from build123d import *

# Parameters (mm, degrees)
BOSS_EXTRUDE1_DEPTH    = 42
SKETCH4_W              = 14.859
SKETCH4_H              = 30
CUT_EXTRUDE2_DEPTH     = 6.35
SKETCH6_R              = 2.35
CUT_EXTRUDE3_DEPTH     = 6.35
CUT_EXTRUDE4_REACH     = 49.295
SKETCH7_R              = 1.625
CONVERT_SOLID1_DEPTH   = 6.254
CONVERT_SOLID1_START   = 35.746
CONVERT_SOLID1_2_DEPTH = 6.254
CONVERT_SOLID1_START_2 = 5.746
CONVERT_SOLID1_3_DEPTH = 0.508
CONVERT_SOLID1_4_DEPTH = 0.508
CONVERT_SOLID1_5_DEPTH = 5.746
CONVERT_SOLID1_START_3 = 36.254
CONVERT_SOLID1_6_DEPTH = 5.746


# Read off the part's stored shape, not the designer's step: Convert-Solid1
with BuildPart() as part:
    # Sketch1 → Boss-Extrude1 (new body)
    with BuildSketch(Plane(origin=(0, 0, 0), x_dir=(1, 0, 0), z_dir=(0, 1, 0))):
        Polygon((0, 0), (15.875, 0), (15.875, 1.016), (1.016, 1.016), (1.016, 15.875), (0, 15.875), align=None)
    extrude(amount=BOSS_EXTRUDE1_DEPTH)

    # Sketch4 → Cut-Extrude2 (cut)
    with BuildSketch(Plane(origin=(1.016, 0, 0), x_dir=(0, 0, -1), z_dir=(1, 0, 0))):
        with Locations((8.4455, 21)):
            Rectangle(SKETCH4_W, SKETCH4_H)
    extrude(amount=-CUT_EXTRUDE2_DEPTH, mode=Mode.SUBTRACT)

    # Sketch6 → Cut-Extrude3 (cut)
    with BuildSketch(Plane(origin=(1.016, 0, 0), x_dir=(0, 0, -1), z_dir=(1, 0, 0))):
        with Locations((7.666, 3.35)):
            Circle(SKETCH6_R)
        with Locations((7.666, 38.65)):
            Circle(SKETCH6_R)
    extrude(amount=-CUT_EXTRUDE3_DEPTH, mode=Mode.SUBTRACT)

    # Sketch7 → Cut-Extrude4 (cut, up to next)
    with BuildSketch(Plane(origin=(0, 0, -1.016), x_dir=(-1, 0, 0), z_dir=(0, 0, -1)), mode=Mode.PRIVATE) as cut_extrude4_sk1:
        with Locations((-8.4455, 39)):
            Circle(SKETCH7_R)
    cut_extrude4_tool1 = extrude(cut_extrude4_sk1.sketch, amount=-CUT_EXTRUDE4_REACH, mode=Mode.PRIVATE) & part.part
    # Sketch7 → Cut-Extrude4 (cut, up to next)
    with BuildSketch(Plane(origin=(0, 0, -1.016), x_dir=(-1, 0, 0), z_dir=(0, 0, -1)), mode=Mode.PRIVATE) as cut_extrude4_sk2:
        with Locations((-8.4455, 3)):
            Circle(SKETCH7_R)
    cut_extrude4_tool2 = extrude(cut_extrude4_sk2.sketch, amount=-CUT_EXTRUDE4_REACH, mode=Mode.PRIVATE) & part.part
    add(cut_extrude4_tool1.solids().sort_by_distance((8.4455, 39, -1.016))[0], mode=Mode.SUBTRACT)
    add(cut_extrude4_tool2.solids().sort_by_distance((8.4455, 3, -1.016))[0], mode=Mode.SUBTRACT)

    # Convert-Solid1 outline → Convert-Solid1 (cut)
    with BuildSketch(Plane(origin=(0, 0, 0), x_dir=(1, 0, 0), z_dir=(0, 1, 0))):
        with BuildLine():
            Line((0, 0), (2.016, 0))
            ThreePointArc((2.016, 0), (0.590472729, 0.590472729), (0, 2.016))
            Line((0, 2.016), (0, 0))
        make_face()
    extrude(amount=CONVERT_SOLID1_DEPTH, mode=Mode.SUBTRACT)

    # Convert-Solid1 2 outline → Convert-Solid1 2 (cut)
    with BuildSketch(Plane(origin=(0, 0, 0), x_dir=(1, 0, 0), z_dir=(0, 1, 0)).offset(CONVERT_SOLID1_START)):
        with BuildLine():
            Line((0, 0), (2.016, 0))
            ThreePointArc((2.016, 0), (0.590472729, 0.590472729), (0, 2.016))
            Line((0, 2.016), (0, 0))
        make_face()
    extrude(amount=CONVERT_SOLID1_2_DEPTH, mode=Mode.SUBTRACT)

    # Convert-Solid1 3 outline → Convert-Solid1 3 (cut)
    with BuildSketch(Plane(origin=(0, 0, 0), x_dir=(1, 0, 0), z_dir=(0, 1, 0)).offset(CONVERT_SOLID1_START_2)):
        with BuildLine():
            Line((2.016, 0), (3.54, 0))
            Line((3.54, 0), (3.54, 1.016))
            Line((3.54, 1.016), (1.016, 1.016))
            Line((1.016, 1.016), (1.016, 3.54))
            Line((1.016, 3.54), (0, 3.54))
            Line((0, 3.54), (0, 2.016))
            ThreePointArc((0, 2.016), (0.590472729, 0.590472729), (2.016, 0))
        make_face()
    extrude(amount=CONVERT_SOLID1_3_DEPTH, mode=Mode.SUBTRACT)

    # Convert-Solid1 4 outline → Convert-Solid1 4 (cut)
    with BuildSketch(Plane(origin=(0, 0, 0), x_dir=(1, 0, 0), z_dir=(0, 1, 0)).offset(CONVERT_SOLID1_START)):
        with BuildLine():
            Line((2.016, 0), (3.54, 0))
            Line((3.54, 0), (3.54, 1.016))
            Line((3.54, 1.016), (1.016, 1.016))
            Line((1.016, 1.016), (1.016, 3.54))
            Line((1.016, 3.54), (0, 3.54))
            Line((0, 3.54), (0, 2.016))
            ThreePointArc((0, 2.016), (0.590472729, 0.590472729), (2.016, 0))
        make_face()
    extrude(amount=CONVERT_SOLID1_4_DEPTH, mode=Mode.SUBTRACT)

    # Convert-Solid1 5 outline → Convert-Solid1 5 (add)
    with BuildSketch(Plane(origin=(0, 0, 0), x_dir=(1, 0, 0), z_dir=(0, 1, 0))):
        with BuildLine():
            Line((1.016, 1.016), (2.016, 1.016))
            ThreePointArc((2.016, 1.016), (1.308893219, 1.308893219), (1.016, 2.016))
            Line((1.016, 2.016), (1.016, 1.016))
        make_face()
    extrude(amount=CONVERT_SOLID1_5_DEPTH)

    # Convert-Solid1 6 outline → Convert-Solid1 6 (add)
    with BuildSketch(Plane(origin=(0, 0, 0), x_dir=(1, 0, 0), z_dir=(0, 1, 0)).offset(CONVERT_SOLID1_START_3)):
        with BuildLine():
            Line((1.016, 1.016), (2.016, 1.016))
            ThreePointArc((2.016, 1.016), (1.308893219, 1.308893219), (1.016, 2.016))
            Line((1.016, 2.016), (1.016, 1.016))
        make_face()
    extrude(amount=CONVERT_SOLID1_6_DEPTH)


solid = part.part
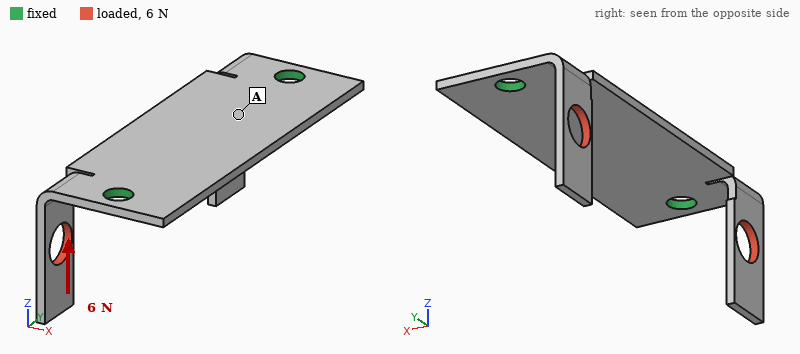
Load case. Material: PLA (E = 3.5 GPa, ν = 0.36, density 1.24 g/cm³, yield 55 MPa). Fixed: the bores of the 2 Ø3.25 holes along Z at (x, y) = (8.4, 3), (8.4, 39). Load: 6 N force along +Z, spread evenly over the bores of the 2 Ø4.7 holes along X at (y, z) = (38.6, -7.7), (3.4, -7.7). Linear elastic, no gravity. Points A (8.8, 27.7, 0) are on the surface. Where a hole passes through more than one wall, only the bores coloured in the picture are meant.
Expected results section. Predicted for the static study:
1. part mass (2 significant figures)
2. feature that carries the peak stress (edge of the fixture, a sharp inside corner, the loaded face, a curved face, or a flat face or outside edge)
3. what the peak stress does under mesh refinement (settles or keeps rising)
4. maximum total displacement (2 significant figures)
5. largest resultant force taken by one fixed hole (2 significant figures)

0.98 g
a sharp inside corner
keeps rising
0.49 mm
3.0 N
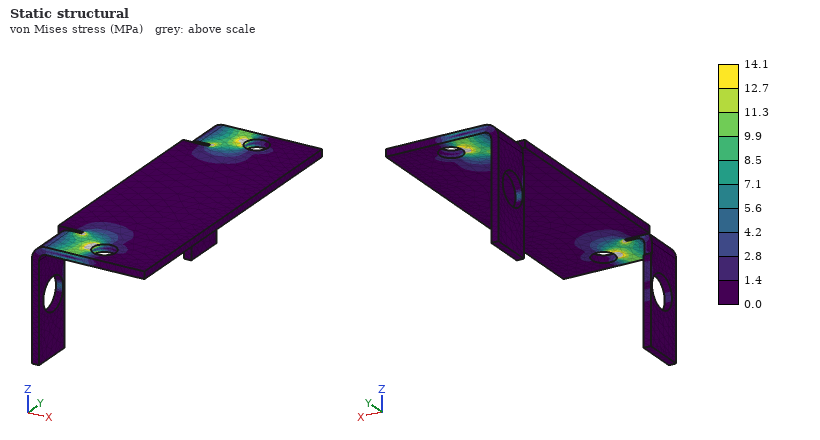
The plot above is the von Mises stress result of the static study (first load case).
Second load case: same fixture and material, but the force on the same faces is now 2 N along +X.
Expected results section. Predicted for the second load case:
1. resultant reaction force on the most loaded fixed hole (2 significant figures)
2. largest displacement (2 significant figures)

1.0 N
0.57 mm
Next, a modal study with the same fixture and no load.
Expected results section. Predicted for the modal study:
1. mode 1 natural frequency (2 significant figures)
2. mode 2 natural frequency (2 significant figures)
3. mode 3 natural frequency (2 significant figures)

700 Hz
710 Hz
1200 Hz
